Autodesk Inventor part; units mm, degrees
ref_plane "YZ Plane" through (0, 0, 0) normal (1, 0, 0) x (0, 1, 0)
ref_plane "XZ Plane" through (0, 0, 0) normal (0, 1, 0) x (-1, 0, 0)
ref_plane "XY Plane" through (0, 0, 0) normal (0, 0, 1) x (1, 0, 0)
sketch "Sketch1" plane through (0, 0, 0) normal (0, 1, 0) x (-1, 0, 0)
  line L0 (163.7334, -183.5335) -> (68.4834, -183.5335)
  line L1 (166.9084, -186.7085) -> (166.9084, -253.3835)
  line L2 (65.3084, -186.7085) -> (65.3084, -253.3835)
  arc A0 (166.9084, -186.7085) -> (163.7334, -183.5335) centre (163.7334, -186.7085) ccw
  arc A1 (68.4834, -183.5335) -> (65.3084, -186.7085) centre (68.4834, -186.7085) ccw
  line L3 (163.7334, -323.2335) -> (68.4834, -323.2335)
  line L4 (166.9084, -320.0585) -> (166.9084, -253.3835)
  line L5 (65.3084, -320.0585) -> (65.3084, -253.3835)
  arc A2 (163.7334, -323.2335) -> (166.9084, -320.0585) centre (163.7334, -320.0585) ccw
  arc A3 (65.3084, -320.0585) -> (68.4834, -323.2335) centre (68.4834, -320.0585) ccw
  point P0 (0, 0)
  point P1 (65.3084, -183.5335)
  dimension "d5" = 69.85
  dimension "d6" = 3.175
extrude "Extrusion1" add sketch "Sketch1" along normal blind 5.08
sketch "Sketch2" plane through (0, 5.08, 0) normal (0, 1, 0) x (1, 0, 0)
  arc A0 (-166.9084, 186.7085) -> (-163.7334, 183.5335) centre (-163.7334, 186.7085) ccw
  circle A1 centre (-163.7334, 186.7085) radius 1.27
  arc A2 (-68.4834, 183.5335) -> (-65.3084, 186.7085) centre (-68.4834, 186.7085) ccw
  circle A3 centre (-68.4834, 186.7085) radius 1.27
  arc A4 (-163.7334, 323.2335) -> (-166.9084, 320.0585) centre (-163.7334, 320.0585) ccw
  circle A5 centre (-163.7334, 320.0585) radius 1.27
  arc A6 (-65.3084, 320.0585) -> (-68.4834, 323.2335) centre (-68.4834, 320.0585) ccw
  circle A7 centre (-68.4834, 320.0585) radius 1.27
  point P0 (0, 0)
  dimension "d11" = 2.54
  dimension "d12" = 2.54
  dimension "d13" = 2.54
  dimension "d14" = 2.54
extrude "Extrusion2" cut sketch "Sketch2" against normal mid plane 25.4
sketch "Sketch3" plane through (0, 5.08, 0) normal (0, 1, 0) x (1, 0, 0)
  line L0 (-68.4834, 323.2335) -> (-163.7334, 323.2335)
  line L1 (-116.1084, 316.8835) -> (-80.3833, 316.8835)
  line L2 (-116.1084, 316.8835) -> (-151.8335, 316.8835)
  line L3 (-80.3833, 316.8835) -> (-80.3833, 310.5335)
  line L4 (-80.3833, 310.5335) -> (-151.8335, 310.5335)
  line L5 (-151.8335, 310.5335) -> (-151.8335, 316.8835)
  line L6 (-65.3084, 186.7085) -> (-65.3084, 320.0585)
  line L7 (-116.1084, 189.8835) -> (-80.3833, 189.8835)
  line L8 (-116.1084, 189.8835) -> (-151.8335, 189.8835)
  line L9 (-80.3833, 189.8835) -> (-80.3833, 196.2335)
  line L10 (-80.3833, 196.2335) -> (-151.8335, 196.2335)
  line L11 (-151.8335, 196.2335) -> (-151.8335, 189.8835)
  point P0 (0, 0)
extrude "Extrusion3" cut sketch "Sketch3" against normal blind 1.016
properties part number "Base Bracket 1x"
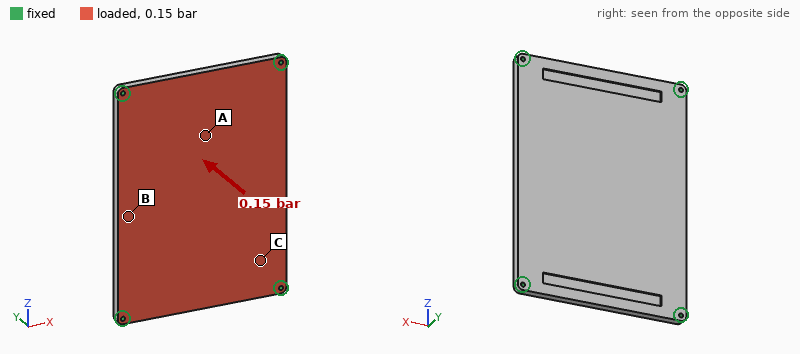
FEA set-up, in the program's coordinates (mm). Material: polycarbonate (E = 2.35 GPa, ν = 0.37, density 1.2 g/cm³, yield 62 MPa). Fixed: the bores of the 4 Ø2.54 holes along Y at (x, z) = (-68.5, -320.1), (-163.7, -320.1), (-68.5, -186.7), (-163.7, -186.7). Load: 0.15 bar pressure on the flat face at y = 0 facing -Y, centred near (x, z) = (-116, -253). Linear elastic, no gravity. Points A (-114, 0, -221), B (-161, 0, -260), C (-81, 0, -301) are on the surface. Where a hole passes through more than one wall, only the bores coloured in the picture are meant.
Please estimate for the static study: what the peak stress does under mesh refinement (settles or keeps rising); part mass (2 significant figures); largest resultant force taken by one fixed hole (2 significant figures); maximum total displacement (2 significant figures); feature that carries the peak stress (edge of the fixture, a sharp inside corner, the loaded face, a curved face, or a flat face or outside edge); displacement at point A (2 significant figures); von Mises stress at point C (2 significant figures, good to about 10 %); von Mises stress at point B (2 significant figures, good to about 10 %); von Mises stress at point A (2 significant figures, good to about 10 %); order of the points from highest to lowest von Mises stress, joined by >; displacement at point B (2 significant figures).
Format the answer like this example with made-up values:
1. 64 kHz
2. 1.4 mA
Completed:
1. keeps rising
2. 85 g
3. 53 N
4. 1.1 mm
5. edge of the fixture
6. 0.87 mm
7. 1.4 MPa
8. 4.3 MPa
9. 2.5 MPa
10. B > A > C
11. 1.0 mm
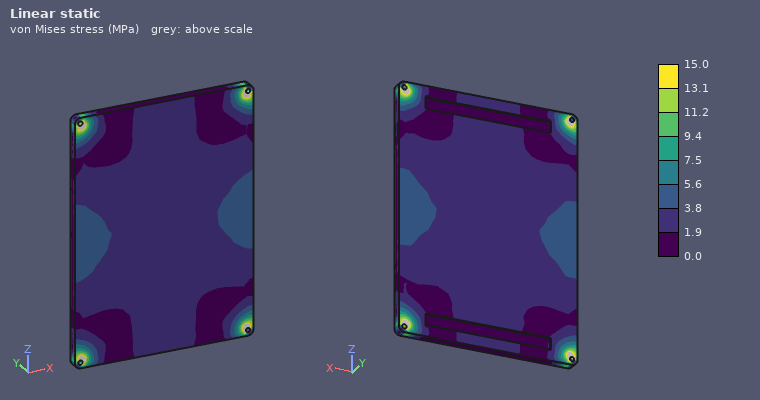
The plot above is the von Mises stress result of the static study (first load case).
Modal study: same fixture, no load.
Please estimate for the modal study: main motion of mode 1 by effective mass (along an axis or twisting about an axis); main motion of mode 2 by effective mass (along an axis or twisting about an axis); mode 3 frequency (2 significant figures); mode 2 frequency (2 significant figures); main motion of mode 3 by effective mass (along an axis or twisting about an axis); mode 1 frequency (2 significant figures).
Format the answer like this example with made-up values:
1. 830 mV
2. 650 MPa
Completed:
1. along Y
2. twisting about Z
3. 640 Hz
4. 480 Hz
5. twisting about X
6. 270 Hz
